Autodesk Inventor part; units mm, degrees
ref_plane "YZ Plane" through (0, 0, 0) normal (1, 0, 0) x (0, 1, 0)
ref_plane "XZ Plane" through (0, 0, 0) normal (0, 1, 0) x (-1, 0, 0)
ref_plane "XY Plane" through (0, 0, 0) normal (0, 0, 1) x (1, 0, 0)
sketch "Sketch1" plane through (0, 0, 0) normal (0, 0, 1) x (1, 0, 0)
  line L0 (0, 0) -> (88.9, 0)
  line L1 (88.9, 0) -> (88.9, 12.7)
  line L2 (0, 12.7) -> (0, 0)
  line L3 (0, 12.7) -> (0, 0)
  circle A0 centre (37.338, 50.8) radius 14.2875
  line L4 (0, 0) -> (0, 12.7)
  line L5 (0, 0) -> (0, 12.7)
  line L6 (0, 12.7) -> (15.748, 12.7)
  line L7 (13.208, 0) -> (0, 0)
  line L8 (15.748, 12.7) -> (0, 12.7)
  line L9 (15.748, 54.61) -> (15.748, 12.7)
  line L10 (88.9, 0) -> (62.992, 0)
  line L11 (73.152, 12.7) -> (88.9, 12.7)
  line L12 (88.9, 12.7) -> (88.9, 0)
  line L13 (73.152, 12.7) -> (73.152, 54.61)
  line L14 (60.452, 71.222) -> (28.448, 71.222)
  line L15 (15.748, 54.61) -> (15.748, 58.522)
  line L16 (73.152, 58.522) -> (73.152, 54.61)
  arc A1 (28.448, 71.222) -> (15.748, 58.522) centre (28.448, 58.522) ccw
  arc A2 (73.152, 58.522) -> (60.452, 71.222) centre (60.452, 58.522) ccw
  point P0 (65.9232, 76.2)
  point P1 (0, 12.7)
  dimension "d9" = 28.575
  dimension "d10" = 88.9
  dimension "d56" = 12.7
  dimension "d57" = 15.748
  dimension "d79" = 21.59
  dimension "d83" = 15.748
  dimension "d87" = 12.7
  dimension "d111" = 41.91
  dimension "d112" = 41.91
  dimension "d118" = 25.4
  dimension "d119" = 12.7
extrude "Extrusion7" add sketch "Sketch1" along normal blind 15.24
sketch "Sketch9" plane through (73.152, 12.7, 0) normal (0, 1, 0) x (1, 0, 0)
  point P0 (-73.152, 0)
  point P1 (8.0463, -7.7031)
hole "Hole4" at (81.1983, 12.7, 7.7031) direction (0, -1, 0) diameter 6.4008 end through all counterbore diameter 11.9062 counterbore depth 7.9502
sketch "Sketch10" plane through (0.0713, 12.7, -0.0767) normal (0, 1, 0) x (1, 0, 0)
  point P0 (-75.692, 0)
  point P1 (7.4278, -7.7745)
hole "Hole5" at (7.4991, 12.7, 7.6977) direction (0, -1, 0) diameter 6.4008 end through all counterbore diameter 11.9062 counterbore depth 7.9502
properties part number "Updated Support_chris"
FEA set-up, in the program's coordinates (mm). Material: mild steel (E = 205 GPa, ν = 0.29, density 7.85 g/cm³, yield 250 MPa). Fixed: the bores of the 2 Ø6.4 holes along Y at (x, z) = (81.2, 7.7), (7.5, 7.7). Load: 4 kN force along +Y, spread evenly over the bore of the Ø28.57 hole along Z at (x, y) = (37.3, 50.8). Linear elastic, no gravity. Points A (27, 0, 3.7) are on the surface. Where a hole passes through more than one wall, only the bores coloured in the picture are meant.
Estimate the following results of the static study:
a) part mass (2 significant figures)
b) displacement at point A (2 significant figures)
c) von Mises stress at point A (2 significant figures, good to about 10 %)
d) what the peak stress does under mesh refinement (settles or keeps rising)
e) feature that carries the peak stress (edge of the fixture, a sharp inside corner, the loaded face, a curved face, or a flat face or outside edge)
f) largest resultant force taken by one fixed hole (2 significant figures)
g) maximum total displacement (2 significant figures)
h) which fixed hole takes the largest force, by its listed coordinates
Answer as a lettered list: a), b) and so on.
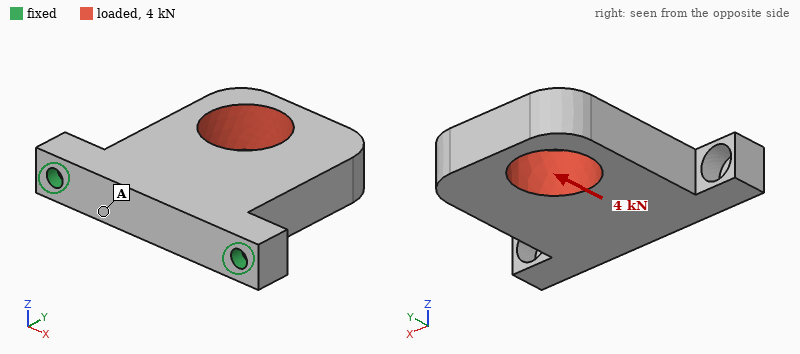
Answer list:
a) 440 g
b) 5.2 µm
c) 12 MPa
d) keeps rising
e) edge of the fixture
f) 2.7 kN
g) 9.3 µm
h) (7.5, 7.7)
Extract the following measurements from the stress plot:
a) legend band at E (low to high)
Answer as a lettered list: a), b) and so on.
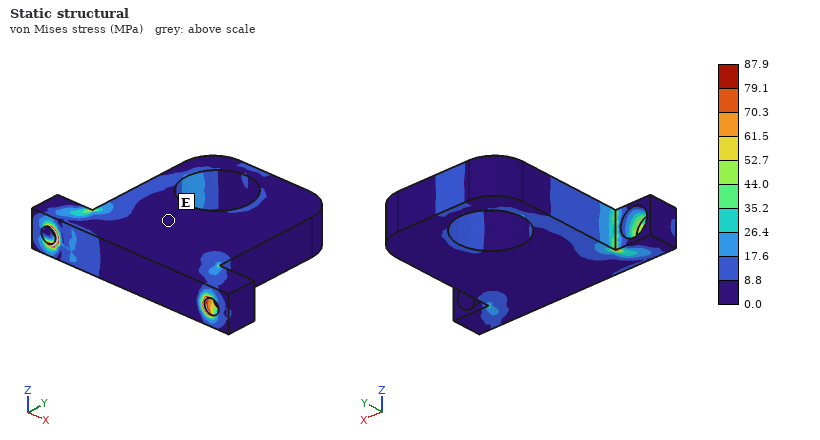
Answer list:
a) 0.0 to 8.8 MPa
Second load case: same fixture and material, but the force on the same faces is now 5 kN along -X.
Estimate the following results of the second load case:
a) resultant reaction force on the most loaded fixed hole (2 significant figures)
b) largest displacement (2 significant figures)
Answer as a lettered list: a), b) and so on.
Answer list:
a) 4.4 kN
b) 28 µm
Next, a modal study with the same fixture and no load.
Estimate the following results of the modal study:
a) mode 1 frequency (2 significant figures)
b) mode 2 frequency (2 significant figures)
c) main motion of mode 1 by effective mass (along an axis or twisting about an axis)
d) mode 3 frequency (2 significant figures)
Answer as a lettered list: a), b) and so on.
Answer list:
a) 1100 Hz
b) 5300 Hz
c) along Z
d) 5400 Hz
